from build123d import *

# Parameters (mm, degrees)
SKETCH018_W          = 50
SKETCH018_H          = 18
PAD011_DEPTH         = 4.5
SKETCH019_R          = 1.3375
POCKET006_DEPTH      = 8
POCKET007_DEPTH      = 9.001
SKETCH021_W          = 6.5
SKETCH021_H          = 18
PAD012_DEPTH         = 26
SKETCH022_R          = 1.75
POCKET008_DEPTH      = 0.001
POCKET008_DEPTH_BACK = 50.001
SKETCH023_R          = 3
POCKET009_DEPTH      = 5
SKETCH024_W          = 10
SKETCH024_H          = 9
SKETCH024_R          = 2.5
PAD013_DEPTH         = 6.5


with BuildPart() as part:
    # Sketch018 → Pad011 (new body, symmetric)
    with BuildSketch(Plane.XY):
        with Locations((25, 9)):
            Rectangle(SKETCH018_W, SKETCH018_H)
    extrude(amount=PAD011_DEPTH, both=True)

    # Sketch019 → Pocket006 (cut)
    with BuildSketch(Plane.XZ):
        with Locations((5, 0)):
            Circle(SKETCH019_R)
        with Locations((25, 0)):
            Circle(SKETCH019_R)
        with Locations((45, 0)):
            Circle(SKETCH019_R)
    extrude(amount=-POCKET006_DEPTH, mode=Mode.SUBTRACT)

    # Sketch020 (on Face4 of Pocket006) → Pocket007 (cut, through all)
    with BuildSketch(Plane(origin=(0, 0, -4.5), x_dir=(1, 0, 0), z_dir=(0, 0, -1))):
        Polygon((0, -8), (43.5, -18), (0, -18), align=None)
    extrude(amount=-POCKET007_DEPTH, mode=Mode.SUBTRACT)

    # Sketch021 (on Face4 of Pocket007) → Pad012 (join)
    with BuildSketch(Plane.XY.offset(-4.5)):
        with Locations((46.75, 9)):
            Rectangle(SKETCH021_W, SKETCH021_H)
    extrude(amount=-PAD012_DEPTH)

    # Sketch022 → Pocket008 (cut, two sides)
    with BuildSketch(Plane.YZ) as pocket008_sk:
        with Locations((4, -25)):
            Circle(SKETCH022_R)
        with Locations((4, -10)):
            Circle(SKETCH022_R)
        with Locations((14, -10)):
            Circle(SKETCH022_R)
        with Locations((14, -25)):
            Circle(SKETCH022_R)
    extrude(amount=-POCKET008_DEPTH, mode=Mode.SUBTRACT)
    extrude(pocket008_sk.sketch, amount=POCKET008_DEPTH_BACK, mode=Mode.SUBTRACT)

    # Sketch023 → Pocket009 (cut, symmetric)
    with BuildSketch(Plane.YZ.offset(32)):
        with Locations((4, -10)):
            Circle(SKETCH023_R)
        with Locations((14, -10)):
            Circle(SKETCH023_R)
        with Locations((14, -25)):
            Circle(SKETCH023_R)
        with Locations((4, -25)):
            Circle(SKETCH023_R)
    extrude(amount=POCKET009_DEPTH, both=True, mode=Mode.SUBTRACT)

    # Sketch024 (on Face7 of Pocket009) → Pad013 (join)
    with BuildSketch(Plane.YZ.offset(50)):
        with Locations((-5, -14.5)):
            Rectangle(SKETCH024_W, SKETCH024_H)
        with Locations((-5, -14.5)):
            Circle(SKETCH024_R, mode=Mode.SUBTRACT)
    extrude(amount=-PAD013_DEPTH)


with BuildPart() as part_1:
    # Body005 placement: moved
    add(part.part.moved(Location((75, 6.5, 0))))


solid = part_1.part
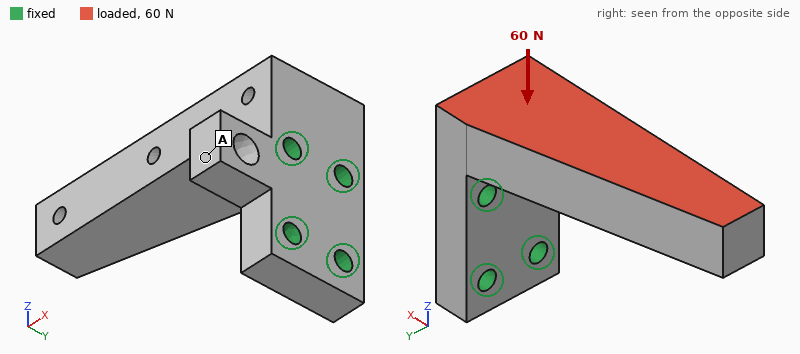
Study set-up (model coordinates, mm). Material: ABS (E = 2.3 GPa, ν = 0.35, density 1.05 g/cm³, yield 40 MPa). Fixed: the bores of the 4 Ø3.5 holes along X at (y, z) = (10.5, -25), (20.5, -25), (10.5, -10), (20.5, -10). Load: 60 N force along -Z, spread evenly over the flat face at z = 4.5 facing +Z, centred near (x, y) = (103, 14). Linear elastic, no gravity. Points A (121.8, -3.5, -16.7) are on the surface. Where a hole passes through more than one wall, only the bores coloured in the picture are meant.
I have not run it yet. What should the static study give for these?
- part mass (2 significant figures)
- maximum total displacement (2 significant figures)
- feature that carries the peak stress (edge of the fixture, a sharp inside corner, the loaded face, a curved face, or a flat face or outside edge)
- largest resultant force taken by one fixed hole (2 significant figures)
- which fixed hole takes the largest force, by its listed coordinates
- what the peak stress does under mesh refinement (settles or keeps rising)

9.7 g
0.67 mm
edge of the fixture
39 N
(10.5, -10)
keeps rising
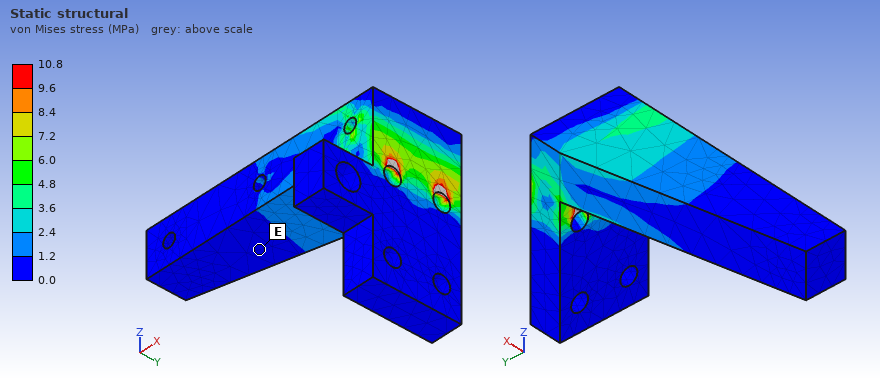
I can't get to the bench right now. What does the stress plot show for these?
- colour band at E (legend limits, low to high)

0.0 to 1.2 MPa
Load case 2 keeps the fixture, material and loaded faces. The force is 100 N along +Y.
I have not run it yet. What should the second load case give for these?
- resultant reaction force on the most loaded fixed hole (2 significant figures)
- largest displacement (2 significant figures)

180 N
0.43 mm
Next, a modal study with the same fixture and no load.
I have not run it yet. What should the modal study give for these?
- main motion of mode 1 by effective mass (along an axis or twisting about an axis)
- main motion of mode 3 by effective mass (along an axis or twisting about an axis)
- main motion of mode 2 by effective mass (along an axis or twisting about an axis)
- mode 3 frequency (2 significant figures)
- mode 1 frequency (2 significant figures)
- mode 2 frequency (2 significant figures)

along Z
along X
along Y
3700 Hz
770 Hz
1200 Hz
